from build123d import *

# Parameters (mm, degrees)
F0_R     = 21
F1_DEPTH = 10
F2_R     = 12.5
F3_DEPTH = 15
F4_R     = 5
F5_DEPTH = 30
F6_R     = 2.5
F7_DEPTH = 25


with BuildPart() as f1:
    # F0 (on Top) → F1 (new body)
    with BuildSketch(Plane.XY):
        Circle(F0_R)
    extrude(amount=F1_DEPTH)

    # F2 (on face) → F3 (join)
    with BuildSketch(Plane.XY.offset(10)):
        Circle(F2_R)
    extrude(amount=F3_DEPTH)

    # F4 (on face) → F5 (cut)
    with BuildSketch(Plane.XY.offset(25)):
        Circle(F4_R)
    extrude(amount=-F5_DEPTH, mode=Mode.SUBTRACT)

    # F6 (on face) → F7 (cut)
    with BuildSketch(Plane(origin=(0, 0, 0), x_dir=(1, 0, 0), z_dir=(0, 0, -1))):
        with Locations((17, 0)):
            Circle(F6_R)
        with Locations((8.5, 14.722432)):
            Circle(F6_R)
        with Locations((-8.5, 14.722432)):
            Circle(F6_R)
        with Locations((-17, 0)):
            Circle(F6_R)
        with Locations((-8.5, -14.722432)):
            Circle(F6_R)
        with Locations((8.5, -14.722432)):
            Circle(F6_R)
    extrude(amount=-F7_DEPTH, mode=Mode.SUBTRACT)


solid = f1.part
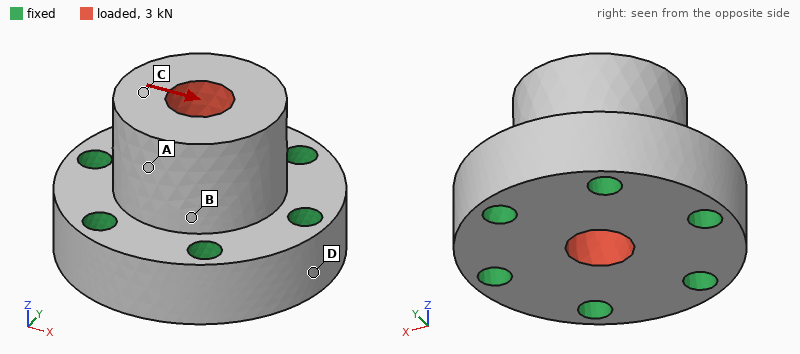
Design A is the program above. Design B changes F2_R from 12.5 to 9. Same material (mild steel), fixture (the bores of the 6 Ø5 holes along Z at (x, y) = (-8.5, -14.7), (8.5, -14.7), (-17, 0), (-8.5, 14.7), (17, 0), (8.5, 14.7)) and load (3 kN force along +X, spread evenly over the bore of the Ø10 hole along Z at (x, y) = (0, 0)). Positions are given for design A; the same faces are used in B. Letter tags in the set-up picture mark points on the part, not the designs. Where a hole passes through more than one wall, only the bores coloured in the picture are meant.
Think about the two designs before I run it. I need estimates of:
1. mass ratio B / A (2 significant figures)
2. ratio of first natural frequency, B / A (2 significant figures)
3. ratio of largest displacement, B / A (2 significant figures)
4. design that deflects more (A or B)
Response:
0.80
0.90
2.8
B
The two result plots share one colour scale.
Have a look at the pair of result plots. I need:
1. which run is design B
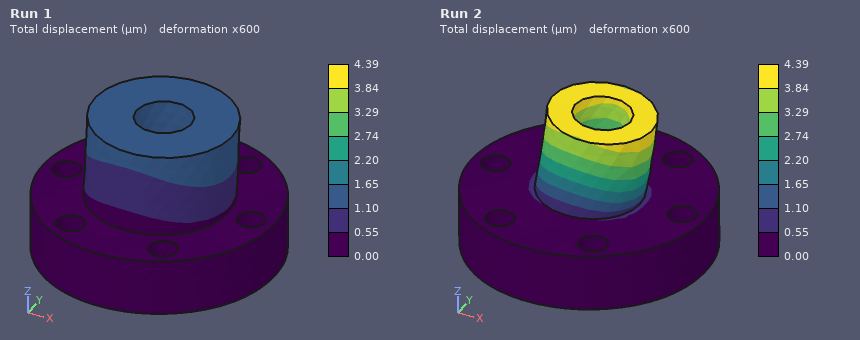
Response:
Run 2
